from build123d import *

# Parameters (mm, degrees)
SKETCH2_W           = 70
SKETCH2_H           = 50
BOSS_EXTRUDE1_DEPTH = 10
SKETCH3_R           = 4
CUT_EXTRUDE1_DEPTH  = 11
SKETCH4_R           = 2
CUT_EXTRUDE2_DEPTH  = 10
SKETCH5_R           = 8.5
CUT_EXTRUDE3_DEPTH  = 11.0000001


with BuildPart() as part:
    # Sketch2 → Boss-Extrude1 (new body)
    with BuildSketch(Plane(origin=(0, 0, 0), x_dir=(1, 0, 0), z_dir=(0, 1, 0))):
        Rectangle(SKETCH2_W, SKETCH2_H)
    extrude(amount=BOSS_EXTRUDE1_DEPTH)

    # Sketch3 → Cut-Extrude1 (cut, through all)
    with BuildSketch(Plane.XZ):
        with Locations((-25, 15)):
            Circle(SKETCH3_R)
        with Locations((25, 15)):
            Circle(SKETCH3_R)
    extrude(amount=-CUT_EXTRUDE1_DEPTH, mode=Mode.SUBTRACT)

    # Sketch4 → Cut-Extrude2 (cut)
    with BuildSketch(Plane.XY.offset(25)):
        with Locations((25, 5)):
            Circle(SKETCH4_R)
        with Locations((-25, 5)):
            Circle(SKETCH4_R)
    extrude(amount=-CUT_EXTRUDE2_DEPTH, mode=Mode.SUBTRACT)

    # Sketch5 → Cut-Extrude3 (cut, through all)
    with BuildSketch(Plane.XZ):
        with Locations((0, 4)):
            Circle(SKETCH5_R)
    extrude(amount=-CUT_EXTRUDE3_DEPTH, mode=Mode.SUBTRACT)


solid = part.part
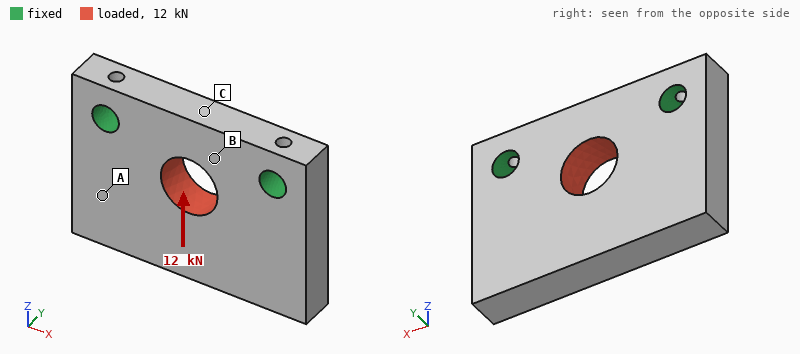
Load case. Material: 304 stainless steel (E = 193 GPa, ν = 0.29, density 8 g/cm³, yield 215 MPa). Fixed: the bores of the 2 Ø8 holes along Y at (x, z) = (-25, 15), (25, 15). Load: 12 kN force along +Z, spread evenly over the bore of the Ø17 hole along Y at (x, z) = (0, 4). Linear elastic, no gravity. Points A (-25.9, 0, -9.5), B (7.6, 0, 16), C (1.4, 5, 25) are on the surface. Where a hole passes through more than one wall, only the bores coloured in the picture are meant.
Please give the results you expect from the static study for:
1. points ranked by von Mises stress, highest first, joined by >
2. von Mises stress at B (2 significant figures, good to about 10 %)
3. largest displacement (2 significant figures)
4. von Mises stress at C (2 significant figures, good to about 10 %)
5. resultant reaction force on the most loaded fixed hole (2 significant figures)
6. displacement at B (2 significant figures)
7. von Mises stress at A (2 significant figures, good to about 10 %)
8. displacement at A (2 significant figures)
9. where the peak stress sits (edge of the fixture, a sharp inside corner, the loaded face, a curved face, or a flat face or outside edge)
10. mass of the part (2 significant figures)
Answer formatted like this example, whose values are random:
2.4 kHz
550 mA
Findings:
C > B > A
25 MPa
6.8 µm
42 MPa
6.2 kN
5.0 µm
11 MPa
1.9 µm
edge of the fixture
250 g
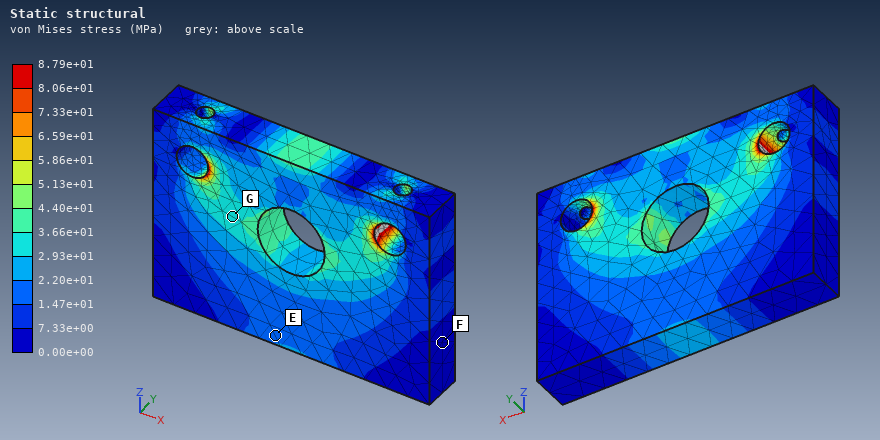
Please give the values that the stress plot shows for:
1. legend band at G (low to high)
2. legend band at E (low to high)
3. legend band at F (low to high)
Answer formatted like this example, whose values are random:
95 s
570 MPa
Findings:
2.93e+01 to 3.66e+01 MPa
1.47e+01 to 2.20e+01 MPa
0.00e+00 to 7.33e+00 MPa
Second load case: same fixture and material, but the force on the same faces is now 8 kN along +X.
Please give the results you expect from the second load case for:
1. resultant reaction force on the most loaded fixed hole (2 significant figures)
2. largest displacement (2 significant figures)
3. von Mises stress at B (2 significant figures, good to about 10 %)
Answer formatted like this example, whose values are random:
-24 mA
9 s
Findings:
4.2 kN
4.5 µm
15 MPa
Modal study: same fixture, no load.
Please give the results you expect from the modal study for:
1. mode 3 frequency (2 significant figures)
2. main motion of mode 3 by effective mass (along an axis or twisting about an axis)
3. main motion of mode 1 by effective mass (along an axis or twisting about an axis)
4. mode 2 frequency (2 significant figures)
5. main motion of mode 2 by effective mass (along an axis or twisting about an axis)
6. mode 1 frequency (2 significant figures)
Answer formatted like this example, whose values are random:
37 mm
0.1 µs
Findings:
13 kHz
along X
along Y
7600 Hz
twisting about Z
4300 Hz
